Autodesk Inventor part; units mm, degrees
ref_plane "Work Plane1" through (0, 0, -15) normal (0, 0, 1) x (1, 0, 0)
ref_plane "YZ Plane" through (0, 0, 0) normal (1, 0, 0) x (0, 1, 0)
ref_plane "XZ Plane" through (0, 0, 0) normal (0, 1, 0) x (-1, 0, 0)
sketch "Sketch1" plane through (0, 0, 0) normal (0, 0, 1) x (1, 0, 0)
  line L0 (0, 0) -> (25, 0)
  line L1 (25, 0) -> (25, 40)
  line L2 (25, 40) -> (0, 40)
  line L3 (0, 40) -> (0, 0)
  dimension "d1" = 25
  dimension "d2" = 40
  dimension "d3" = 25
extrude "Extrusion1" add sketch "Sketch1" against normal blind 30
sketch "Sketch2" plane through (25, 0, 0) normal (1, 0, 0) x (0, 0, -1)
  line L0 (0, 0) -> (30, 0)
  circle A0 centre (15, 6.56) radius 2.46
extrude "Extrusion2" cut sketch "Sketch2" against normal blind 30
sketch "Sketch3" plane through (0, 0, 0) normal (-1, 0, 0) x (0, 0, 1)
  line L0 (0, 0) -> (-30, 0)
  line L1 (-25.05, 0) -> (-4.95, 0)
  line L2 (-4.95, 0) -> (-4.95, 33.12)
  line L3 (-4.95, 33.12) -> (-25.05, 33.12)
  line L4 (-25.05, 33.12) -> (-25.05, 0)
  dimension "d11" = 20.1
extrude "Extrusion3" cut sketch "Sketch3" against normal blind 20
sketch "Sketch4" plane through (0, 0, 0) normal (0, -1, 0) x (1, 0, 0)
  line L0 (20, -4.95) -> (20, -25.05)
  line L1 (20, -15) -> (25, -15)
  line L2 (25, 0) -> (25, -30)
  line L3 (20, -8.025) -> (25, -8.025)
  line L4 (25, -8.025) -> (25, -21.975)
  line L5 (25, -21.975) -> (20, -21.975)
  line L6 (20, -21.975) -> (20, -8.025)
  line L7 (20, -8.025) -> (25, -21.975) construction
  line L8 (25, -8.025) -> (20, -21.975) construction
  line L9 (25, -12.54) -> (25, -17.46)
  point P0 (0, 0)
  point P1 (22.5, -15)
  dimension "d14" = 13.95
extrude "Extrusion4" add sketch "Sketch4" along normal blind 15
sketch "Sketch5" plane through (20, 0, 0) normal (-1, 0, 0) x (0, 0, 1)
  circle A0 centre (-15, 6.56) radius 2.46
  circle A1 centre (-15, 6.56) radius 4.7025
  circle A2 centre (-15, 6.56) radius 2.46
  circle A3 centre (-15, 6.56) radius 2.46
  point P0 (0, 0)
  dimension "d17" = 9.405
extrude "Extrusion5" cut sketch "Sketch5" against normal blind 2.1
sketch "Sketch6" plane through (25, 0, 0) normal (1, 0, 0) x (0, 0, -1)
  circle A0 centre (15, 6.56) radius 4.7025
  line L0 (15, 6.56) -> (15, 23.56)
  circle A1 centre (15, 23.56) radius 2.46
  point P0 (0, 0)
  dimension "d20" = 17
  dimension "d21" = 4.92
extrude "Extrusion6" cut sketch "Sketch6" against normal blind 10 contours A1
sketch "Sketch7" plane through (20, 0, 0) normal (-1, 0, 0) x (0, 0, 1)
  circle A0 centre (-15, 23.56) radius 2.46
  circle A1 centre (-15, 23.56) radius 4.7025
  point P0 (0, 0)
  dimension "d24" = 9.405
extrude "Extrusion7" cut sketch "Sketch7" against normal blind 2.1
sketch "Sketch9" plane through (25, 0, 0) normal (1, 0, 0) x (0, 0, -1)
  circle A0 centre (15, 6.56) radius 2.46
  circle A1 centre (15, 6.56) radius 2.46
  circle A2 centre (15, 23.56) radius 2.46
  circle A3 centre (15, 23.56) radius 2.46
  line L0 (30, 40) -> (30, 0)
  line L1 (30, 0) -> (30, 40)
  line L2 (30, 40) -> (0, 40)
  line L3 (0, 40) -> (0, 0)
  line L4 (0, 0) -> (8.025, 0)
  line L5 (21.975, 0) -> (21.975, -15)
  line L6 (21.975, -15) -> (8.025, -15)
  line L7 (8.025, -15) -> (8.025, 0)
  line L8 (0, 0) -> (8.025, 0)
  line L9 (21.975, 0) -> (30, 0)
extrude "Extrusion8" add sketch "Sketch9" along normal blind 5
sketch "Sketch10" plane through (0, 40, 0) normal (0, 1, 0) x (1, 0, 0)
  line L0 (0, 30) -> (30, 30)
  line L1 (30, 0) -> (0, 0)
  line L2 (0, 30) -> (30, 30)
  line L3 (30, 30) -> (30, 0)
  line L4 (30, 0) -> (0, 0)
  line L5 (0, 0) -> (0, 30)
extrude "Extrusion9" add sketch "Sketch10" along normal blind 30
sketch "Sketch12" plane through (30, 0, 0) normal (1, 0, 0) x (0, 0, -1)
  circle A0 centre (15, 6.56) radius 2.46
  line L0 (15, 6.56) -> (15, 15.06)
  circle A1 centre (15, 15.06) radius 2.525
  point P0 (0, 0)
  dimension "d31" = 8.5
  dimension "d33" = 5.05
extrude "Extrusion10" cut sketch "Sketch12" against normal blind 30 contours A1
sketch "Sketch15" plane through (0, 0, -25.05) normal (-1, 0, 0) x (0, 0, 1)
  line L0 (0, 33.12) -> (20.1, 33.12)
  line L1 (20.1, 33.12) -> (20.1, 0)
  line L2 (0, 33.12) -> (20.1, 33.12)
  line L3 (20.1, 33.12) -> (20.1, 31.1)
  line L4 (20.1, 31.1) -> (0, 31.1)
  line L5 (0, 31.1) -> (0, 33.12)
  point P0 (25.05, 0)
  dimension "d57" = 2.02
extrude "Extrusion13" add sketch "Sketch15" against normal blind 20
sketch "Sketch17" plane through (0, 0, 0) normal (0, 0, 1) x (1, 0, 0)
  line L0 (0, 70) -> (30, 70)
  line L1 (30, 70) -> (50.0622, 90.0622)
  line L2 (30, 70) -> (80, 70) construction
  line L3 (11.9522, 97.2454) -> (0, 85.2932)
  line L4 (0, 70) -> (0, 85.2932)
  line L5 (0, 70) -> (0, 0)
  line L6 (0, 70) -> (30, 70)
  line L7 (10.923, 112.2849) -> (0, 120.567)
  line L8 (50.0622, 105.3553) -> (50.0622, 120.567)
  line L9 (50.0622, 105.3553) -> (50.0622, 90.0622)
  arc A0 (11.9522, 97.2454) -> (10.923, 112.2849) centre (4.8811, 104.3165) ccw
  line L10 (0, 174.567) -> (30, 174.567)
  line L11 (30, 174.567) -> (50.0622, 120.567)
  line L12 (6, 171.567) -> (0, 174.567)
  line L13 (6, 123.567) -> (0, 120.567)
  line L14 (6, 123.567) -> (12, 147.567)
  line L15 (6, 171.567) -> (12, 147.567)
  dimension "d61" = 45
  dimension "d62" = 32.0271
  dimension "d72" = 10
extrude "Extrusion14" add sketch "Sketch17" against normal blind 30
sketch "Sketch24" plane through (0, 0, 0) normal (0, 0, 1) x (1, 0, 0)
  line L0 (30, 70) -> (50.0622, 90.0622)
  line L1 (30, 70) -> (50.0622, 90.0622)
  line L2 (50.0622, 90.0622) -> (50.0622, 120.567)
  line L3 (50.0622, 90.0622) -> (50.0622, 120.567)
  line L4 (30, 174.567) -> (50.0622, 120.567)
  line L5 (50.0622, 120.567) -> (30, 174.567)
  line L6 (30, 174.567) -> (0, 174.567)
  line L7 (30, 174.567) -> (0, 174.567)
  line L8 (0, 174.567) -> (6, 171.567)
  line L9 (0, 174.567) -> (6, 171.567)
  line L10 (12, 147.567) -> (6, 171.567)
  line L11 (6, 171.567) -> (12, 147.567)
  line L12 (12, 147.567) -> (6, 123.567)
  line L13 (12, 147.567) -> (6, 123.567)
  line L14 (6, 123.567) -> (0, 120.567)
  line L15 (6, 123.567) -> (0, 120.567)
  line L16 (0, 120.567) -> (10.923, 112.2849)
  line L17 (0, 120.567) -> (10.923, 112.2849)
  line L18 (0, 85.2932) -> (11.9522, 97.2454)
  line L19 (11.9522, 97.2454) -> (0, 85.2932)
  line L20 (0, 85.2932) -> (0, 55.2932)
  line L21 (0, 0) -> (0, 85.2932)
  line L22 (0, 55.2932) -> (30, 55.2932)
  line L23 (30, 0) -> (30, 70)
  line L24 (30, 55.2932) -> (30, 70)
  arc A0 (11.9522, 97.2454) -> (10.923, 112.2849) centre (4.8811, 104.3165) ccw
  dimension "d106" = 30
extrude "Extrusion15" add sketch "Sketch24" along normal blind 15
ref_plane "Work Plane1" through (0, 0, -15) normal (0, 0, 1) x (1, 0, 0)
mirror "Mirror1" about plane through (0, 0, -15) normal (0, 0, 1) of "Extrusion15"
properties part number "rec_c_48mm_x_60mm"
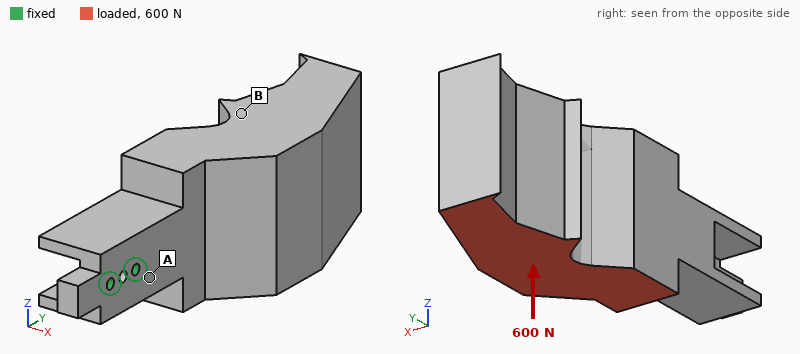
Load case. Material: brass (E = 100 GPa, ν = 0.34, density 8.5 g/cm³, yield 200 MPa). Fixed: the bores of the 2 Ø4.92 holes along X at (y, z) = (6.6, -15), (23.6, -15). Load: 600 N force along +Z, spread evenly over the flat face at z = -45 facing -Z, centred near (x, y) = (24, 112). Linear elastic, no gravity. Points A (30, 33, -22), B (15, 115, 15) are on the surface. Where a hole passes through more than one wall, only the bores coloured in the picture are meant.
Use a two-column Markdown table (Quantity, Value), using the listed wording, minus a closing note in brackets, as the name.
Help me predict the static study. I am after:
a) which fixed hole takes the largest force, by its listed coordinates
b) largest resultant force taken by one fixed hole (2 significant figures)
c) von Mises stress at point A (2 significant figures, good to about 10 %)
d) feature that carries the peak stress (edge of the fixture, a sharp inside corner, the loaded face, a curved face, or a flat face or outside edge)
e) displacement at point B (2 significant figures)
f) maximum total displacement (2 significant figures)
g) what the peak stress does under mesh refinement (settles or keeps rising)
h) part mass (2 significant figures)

| Quantity | Value |
|---|---|
| which fixed hole takes the largest force, by its listed coordinates | (23.6, -15) |
| largest resultant force taken by one fixed hole | 2.9 kN |
| von Mises stress at point A | 12 MPa |
| feature that carries the peak stress | edge of the fixture |
| displacement at point B | 0.070 mm |
| maximum total displacement | 0.12 mm |
| what the peak stress does under mesh refinement | keeps rising |
| part mass | 2.4 kg |
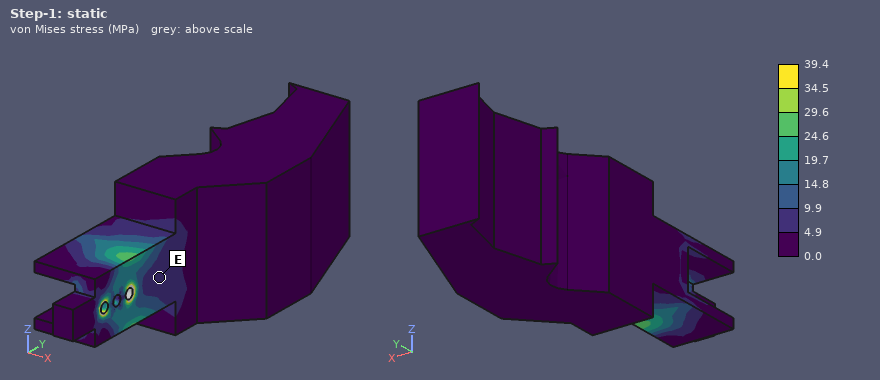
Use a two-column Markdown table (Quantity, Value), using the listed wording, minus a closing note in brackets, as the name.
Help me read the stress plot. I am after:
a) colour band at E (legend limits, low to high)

| Quantity | Value |
|---|---|
| colour band at E | 4.9 to 9.9 MPa |
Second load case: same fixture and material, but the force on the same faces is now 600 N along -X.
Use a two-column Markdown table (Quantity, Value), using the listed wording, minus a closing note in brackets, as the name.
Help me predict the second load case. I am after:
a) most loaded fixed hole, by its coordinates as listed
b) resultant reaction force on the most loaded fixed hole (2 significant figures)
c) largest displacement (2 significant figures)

| Quantity | Value |
|---|---|
| most loaded fixed hole, by its coordinates as listed | (23.6, -15) |
| resultant reaction force on the most loaded fixed hole | 2.7 kN |
| largest displacement | 0.18 mm |
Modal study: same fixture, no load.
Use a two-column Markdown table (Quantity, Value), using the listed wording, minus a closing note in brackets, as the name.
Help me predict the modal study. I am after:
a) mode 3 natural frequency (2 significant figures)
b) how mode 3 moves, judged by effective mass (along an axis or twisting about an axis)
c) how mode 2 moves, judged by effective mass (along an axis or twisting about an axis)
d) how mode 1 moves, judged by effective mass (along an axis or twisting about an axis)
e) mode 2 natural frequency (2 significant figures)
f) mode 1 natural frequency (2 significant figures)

| Quantity | Value |
|---|---|
| mode 3 natural frequency | 810 Hz |
| how mode 3 moves, judged by effective mass | twisting about Y |
| how mode 2 moves, judged by effective mass | along Z |
| how mode 1 moves, judged by effective mass | along X |
| mode 2 natural frequency | 300 Hz |
| mode 1 natural frequency | 260 Hz |
